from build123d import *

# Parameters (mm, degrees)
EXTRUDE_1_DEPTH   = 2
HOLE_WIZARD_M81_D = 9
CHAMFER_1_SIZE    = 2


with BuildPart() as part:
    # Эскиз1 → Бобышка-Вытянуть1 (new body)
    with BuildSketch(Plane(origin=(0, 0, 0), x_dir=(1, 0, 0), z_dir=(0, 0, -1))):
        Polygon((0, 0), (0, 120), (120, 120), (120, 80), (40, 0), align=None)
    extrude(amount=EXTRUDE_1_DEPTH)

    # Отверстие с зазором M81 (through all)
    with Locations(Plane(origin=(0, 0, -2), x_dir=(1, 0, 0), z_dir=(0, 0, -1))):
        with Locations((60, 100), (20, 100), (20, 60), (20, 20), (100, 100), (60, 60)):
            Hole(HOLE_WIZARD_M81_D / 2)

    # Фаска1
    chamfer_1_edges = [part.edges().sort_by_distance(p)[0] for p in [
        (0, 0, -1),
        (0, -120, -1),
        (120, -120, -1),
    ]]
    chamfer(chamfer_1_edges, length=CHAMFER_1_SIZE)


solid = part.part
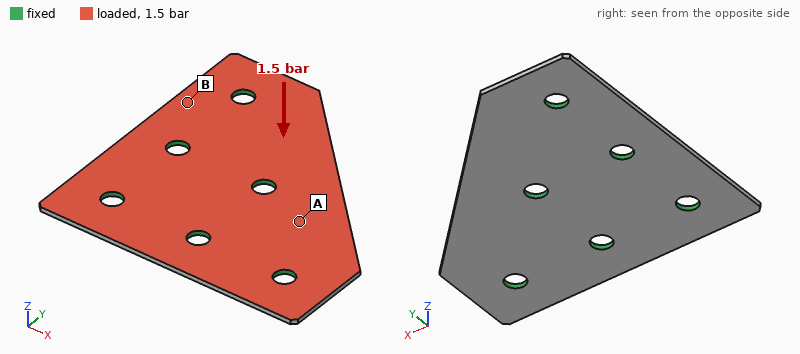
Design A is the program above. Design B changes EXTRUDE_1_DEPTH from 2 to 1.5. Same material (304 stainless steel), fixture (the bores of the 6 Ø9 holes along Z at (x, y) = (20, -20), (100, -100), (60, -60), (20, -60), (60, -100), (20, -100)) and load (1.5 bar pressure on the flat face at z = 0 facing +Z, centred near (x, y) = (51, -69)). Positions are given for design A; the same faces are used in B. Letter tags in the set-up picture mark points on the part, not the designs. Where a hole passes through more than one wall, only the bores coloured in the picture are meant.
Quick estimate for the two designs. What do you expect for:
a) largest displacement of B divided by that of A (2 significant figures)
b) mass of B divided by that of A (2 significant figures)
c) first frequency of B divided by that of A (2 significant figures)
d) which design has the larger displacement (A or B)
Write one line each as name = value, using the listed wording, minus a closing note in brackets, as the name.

largest displacement of B divided by that of A = 2.3
mass of B divided by that of A = 0.75
first frequency of B divided by that of A = 0.75
which design has the larger displacement = B
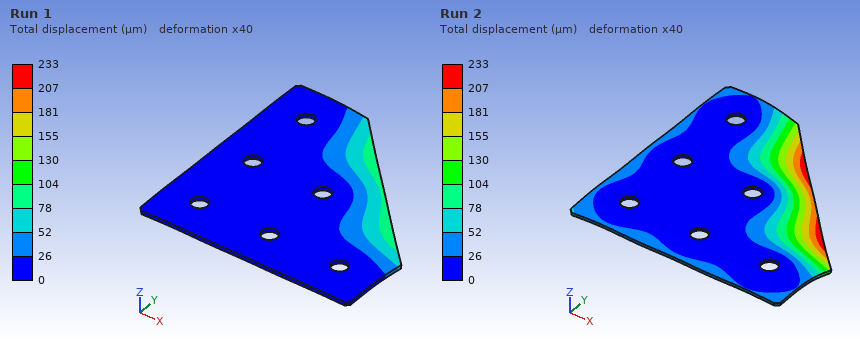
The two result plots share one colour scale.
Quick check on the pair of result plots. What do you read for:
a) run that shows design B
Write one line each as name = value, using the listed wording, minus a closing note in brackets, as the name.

run that shows design B = Run 2
